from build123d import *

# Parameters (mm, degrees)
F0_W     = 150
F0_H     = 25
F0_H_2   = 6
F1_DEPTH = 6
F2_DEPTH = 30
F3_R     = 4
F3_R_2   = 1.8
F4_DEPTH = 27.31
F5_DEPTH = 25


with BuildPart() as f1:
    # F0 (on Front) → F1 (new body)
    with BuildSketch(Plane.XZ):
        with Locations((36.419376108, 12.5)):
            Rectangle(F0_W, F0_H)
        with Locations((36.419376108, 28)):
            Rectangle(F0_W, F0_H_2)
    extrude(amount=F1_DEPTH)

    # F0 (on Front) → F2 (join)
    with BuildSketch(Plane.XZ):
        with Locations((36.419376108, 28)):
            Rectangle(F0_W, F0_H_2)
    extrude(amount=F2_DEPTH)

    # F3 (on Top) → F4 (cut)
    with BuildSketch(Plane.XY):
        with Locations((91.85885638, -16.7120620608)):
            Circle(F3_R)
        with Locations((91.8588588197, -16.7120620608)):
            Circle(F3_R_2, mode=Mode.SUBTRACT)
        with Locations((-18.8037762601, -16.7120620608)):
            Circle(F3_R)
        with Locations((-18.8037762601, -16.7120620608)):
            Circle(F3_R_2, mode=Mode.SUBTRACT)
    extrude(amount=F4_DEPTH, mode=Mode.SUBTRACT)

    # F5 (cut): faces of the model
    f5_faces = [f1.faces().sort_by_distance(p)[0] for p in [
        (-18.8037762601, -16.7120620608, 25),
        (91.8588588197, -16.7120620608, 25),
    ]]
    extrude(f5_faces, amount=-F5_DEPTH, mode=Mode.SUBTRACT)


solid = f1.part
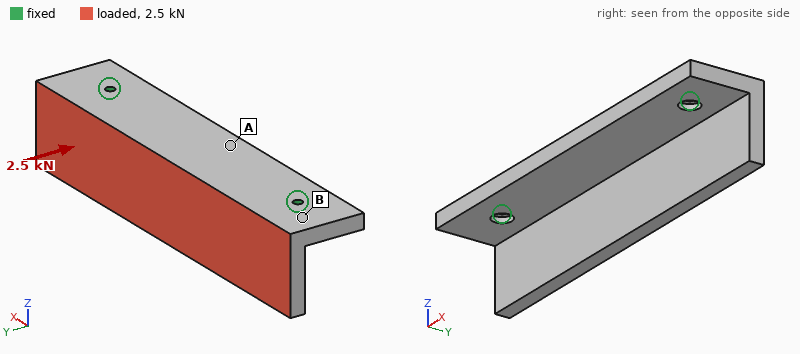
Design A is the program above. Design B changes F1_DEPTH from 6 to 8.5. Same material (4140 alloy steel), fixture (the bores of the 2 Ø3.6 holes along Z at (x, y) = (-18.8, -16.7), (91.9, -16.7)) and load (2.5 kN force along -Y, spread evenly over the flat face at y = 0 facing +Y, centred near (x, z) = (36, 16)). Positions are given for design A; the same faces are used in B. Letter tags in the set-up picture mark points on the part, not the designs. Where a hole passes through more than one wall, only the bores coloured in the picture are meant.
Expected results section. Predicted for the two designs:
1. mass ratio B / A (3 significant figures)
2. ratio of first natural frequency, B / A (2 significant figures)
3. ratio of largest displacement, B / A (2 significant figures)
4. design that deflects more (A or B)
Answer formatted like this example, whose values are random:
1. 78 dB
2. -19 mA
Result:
1. 1.19
2. 0.90
3. 0.89
4. A
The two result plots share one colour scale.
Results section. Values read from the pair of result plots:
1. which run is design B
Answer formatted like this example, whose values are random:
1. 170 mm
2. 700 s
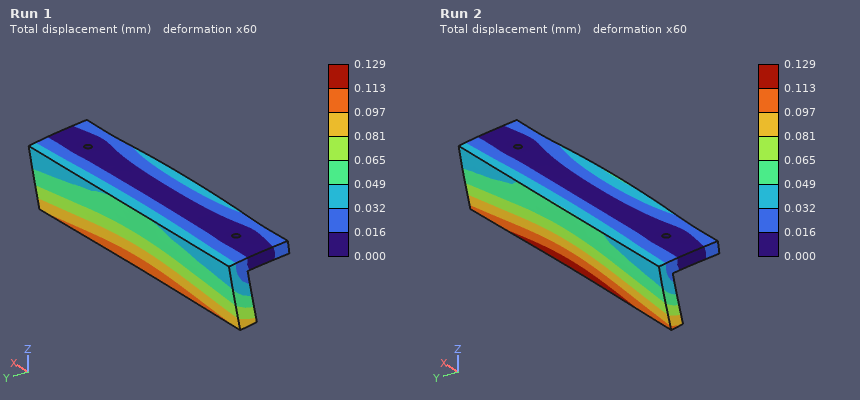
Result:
1. Run 1
